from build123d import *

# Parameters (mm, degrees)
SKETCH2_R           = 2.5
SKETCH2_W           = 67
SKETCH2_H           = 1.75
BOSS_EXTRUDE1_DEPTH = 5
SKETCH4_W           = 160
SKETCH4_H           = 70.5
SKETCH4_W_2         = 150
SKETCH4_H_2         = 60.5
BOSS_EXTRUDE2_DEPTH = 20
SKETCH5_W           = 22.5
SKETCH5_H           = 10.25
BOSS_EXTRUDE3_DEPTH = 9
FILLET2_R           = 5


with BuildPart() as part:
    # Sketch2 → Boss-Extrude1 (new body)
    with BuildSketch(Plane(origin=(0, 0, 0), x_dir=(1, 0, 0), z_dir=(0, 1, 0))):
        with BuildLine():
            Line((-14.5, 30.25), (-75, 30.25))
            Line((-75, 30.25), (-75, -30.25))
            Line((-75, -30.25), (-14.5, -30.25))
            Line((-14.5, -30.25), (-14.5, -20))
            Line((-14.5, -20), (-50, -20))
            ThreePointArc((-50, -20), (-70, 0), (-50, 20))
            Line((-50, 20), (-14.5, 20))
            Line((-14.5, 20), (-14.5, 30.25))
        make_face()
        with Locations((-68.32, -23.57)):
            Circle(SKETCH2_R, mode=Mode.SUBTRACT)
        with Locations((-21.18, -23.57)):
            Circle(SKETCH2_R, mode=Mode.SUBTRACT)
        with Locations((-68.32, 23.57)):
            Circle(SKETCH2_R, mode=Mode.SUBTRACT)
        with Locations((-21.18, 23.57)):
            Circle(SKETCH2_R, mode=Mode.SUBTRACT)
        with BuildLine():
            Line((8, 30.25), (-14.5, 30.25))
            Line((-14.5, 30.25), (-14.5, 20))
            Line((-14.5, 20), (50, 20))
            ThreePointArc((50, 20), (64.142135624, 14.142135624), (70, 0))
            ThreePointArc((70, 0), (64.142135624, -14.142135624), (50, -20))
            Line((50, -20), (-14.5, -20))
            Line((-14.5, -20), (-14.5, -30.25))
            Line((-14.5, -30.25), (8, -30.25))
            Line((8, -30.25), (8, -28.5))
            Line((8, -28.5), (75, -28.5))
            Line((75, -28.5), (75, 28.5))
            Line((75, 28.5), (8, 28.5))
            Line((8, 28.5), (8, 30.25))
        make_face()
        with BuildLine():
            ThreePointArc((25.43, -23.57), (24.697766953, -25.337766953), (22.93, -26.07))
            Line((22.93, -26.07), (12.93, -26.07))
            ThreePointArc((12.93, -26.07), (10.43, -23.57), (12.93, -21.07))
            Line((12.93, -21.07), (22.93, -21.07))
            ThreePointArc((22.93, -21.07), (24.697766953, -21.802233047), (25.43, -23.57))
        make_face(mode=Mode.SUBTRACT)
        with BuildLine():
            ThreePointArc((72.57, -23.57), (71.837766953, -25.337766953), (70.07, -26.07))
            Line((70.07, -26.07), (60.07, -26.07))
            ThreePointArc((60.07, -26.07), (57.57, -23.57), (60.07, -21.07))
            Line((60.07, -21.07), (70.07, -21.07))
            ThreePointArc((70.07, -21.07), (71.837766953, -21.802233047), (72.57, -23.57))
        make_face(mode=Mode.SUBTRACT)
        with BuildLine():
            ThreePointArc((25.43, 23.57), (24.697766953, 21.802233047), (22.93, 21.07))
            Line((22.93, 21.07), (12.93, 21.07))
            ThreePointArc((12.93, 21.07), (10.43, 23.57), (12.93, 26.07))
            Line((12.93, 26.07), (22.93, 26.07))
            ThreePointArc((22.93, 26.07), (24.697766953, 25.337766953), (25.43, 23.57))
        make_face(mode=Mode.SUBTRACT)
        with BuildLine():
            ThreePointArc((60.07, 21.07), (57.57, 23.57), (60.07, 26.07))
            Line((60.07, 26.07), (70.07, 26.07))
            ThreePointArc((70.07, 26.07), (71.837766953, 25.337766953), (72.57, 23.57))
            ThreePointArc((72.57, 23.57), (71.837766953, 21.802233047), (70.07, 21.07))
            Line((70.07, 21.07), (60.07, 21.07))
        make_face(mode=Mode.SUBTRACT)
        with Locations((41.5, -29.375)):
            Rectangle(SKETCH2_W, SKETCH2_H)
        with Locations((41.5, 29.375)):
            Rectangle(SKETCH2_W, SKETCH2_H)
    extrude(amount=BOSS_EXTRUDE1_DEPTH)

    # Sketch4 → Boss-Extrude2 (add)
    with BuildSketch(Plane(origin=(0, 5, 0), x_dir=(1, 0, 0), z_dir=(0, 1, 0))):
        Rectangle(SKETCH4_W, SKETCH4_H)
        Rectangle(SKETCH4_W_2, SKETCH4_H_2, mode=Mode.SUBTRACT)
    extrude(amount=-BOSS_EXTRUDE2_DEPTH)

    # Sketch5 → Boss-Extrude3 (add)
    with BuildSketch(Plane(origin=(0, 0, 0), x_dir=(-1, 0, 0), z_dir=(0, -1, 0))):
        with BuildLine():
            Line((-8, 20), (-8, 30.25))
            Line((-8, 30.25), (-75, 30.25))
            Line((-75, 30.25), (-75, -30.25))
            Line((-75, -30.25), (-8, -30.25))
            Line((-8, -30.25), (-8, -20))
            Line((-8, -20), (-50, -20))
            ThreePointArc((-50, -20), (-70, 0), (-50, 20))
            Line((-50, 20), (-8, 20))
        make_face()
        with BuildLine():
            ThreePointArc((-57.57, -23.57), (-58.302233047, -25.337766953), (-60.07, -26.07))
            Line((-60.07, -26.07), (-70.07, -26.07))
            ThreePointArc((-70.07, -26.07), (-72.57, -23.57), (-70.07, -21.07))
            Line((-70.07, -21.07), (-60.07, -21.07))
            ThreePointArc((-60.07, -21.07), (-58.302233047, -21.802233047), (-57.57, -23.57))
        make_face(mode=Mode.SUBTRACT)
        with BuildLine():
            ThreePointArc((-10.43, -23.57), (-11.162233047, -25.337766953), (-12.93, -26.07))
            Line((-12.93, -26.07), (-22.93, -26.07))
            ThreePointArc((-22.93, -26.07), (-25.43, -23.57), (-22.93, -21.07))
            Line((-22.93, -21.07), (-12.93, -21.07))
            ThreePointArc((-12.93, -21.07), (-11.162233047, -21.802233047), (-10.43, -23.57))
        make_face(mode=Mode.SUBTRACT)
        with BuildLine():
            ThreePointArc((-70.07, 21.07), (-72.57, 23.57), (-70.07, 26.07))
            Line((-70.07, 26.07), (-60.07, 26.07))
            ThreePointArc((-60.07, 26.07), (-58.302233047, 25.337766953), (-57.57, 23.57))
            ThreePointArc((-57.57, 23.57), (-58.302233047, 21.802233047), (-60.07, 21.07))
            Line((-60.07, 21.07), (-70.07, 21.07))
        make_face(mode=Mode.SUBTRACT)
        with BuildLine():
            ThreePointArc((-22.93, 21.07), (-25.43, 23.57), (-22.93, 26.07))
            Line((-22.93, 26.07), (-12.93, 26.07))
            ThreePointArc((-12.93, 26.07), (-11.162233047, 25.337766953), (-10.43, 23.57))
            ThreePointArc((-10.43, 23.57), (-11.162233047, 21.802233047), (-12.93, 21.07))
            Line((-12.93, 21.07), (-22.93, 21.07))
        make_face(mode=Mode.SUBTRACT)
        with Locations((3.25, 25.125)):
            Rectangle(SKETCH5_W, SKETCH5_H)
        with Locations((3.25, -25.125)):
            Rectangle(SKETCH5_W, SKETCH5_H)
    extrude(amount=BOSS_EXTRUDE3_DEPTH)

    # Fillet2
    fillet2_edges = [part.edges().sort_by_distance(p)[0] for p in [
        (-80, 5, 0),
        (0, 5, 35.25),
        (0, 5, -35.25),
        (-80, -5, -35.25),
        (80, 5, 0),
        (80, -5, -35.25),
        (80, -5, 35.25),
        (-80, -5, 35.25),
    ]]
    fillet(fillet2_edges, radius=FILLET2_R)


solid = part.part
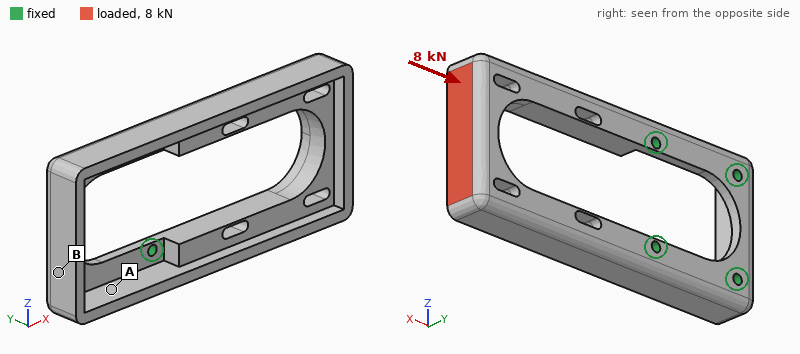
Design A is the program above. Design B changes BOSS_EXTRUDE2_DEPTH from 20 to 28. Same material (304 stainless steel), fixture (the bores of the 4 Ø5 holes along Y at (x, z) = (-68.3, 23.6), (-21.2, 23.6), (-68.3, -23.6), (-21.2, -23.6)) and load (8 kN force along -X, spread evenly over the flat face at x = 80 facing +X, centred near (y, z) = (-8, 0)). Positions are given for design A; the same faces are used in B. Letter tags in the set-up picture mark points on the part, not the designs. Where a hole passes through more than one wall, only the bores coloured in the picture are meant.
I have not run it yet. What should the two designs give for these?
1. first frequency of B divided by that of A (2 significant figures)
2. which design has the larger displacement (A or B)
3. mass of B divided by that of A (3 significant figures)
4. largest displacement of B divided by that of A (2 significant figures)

1.2
A
1.23
0.87
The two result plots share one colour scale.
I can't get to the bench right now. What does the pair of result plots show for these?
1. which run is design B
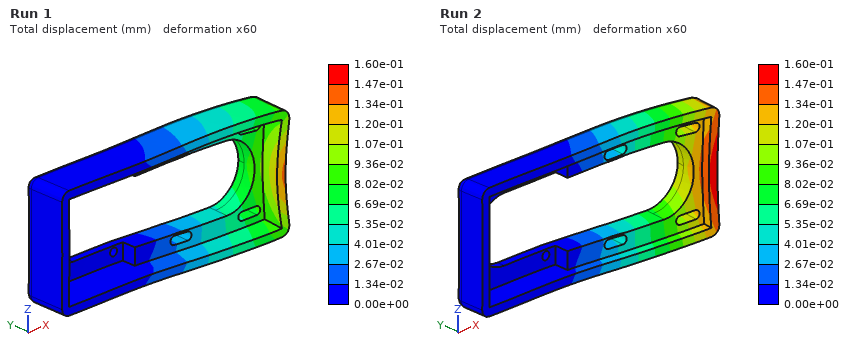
Run 1
